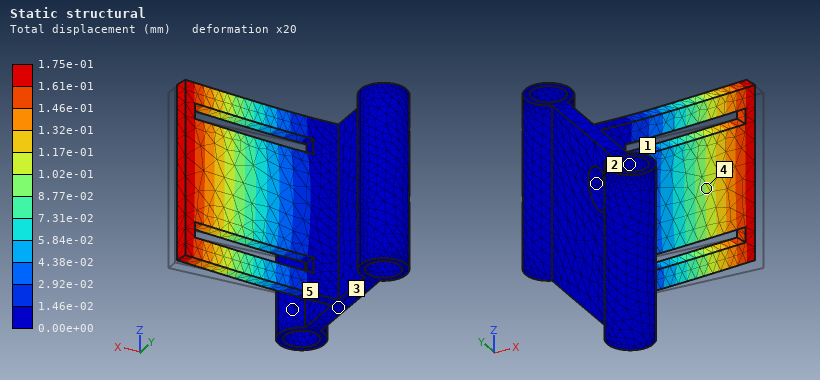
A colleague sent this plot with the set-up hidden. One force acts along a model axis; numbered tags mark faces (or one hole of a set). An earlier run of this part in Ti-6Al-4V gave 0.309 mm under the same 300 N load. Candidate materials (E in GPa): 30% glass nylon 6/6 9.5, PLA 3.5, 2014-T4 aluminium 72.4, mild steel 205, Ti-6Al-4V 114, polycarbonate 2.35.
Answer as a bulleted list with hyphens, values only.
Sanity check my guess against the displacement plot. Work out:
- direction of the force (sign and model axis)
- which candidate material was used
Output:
- +Y
- mild steel
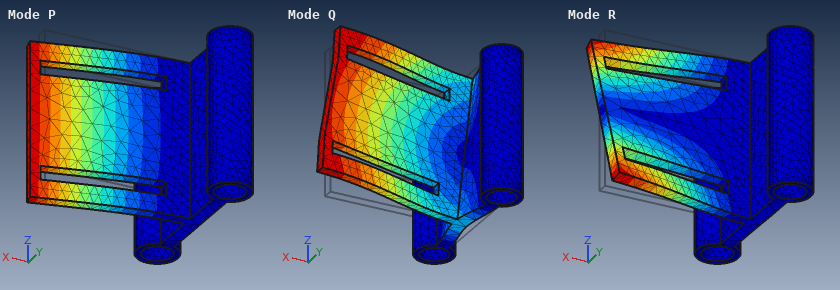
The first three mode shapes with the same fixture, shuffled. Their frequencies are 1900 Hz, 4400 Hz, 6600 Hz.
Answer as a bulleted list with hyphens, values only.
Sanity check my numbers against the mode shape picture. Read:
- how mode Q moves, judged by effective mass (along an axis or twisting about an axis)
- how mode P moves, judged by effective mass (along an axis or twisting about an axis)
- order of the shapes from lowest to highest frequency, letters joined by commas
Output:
- along Z
- along Y
- P, R, Q
